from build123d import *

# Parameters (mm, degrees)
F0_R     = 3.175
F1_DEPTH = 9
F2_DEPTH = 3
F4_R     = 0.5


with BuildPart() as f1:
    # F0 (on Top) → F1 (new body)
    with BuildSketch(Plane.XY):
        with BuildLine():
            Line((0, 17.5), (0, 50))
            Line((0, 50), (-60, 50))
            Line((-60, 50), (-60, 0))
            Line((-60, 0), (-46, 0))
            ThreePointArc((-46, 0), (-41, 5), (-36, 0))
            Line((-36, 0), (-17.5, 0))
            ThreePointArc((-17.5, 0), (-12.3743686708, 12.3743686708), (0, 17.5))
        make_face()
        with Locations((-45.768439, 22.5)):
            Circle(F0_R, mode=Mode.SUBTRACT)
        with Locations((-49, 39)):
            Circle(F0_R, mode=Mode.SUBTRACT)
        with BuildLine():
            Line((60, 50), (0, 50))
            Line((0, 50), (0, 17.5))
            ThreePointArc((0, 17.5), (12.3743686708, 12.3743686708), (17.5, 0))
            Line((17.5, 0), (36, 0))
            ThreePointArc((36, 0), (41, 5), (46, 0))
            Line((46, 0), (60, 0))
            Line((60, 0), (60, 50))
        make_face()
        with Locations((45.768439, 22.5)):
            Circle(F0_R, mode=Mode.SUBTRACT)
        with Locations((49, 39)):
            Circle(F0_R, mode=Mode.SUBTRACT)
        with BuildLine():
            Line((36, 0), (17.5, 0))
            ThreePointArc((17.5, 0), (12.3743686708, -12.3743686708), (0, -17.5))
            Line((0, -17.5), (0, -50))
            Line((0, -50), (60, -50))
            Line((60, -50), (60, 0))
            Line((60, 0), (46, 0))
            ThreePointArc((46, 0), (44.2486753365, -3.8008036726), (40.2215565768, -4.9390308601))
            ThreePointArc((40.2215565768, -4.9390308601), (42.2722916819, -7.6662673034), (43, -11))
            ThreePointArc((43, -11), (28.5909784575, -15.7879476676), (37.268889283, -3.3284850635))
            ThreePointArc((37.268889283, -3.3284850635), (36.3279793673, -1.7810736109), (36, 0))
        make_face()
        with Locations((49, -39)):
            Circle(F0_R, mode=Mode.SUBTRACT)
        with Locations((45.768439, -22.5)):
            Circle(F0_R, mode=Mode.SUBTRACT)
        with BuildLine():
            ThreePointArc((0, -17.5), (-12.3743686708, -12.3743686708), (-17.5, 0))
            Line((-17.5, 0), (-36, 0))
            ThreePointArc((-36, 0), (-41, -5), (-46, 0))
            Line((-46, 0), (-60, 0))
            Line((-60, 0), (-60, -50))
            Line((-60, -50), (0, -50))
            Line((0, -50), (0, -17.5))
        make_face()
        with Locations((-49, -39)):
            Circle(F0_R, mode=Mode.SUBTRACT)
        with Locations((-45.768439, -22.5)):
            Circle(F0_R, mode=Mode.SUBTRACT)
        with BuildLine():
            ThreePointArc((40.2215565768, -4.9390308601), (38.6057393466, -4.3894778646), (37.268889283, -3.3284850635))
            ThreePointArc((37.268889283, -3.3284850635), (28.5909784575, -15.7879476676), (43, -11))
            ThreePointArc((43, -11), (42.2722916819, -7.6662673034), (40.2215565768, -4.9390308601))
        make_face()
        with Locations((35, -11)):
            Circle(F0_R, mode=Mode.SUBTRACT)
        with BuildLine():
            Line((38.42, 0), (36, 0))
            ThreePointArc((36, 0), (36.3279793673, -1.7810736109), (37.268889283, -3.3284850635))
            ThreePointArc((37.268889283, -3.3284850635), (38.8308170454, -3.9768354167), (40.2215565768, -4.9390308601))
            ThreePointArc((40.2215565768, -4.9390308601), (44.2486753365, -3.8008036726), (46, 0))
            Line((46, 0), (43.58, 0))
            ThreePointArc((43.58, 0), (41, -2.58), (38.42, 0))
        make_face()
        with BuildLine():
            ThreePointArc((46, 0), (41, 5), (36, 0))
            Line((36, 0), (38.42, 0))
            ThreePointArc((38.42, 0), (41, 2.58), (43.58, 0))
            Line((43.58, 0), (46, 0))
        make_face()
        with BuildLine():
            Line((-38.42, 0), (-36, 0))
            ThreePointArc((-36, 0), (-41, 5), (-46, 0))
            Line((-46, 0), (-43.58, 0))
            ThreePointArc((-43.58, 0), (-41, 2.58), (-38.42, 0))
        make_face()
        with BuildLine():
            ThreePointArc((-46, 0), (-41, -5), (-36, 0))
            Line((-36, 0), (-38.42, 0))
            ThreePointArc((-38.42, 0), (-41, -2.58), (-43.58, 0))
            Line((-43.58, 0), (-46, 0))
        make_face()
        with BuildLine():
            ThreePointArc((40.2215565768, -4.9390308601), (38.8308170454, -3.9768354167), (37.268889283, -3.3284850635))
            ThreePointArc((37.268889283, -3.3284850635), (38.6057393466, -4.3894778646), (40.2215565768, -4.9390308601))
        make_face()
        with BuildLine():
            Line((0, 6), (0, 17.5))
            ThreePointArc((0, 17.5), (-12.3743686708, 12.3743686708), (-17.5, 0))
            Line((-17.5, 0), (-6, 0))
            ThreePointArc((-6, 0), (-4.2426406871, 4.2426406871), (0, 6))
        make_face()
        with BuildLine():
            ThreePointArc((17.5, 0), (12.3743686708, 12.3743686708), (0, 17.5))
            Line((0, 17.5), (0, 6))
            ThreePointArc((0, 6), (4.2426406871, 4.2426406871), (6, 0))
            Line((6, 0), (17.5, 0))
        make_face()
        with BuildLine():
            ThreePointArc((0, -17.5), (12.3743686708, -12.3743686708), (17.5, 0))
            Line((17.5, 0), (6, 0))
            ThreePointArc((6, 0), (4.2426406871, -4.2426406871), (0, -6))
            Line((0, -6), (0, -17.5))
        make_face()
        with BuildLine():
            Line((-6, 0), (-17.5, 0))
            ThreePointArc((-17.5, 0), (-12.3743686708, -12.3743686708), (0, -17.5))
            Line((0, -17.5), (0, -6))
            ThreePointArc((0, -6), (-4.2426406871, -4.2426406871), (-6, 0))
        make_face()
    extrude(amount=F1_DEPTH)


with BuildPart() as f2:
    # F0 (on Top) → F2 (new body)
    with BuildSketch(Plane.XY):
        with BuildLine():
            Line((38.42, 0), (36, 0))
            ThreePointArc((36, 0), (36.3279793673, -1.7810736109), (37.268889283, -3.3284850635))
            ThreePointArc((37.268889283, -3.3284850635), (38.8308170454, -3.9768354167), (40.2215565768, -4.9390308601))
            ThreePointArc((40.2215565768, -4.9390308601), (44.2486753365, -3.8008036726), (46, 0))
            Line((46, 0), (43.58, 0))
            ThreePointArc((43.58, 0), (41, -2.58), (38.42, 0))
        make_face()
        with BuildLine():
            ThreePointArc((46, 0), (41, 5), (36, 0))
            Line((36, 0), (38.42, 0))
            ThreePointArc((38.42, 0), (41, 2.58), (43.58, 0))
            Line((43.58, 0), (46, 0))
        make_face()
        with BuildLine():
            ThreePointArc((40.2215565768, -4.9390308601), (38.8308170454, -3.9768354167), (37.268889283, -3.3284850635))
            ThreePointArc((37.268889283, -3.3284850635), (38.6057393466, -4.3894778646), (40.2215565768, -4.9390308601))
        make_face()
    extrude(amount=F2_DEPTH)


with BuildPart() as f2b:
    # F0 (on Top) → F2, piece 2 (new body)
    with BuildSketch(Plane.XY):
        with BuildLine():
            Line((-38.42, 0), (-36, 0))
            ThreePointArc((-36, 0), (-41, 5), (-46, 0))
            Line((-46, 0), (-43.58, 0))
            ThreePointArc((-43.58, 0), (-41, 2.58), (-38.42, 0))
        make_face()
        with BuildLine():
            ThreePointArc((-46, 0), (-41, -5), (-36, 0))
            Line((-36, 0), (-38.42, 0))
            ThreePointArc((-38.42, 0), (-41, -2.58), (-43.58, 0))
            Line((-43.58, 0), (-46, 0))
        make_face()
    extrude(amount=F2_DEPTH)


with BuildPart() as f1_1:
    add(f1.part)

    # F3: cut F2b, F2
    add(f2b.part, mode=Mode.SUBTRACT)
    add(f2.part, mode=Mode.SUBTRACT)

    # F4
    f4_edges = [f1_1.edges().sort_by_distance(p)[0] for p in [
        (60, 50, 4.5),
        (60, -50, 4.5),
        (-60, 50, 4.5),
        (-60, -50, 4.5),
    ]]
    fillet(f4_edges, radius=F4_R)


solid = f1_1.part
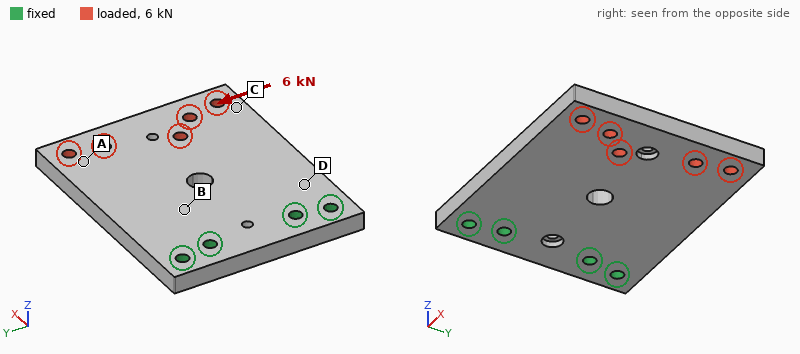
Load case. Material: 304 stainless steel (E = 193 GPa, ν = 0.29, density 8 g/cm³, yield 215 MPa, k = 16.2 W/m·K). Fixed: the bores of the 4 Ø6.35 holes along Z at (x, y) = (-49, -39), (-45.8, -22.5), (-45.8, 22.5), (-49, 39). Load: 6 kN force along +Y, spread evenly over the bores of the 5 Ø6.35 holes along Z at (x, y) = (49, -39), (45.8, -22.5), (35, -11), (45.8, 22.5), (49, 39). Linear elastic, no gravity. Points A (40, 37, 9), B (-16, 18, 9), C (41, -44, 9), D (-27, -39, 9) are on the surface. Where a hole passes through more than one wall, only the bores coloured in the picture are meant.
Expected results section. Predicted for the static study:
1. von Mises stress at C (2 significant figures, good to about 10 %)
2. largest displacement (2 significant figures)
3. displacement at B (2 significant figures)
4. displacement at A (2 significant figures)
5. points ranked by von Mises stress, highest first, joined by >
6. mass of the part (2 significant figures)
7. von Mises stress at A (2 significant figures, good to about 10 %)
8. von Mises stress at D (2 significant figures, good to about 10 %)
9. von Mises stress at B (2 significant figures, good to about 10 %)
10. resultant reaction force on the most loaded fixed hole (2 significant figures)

5.0 MPa
28 µm
5.4 µm
22 µm
D > B > A > C
830 g
9.6 MPa
24 MPa
16 MPa
5.5 kN
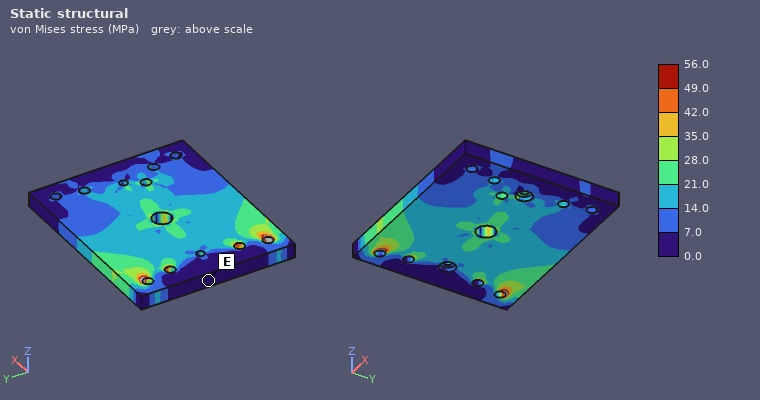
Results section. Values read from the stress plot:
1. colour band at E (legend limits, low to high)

0.0 to 7.0 MPa
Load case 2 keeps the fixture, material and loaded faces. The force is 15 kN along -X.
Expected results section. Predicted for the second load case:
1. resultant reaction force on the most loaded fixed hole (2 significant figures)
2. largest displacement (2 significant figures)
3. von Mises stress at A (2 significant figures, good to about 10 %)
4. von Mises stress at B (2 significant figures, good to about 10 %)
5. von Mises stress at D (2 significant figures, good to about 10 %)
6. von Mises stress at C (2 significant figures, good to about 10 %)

4.4 kN
11 µm
18 MPa
18 MPa
20 MPa
17 MPa
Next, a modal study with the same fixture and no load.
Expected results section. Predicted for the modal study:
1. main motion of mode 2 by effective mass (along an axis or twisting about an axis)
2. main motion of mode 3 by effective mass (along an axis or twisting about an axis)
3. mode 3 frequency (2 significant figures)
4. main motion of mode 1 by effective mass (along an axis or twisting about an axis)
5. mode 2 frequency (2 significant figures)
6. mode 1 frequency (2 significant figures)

twisting about X
along Z
3700 Hz
along Z
1600 Hz
630 Hz
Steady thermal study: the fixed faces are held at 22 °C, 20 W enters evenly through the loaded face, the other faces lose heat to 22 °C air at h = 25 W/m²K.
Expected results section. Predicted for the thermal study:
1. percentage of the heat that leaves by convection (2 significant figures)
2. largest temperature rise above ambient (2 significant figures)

77 %
58 K
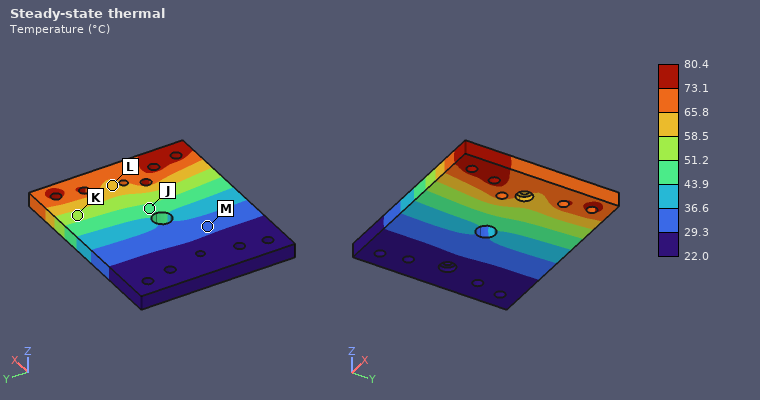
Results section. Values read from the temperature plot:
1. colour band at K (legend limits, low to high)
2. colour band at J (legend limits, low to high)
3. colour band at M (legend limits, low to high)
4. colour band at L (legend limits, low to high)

51.2 to 58.5 °C
43.9 to 51.2 °C
29.3 to 36.6 °C
58.5 to 65.8 °C
